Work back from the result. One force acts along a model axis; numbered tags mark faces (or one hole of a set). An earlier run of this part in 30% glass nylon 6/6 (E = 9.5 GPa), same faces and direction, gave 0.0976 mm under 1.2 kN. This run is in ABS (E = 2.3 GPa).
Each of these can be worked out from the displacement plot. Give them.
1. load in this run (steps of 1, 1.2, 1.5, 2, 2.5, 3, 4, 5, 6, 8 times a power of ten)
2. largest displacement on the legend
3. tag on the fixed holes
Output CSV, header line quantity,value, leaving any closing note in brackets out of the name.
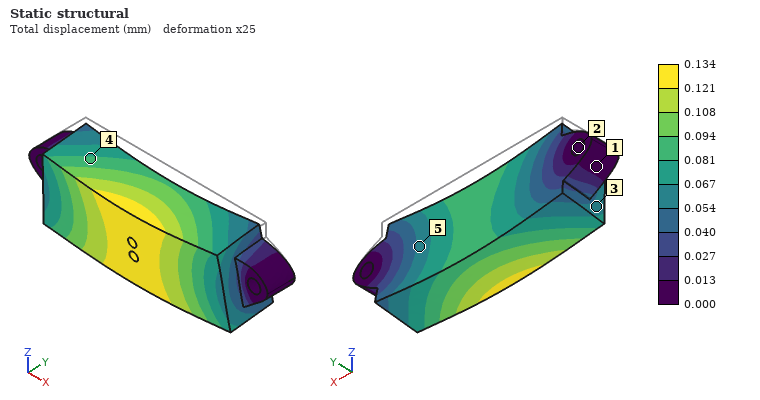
quantity,value
load in this run,400 N
largest displacement on the legend,0.134 mm
tag on the fixed holes,2
